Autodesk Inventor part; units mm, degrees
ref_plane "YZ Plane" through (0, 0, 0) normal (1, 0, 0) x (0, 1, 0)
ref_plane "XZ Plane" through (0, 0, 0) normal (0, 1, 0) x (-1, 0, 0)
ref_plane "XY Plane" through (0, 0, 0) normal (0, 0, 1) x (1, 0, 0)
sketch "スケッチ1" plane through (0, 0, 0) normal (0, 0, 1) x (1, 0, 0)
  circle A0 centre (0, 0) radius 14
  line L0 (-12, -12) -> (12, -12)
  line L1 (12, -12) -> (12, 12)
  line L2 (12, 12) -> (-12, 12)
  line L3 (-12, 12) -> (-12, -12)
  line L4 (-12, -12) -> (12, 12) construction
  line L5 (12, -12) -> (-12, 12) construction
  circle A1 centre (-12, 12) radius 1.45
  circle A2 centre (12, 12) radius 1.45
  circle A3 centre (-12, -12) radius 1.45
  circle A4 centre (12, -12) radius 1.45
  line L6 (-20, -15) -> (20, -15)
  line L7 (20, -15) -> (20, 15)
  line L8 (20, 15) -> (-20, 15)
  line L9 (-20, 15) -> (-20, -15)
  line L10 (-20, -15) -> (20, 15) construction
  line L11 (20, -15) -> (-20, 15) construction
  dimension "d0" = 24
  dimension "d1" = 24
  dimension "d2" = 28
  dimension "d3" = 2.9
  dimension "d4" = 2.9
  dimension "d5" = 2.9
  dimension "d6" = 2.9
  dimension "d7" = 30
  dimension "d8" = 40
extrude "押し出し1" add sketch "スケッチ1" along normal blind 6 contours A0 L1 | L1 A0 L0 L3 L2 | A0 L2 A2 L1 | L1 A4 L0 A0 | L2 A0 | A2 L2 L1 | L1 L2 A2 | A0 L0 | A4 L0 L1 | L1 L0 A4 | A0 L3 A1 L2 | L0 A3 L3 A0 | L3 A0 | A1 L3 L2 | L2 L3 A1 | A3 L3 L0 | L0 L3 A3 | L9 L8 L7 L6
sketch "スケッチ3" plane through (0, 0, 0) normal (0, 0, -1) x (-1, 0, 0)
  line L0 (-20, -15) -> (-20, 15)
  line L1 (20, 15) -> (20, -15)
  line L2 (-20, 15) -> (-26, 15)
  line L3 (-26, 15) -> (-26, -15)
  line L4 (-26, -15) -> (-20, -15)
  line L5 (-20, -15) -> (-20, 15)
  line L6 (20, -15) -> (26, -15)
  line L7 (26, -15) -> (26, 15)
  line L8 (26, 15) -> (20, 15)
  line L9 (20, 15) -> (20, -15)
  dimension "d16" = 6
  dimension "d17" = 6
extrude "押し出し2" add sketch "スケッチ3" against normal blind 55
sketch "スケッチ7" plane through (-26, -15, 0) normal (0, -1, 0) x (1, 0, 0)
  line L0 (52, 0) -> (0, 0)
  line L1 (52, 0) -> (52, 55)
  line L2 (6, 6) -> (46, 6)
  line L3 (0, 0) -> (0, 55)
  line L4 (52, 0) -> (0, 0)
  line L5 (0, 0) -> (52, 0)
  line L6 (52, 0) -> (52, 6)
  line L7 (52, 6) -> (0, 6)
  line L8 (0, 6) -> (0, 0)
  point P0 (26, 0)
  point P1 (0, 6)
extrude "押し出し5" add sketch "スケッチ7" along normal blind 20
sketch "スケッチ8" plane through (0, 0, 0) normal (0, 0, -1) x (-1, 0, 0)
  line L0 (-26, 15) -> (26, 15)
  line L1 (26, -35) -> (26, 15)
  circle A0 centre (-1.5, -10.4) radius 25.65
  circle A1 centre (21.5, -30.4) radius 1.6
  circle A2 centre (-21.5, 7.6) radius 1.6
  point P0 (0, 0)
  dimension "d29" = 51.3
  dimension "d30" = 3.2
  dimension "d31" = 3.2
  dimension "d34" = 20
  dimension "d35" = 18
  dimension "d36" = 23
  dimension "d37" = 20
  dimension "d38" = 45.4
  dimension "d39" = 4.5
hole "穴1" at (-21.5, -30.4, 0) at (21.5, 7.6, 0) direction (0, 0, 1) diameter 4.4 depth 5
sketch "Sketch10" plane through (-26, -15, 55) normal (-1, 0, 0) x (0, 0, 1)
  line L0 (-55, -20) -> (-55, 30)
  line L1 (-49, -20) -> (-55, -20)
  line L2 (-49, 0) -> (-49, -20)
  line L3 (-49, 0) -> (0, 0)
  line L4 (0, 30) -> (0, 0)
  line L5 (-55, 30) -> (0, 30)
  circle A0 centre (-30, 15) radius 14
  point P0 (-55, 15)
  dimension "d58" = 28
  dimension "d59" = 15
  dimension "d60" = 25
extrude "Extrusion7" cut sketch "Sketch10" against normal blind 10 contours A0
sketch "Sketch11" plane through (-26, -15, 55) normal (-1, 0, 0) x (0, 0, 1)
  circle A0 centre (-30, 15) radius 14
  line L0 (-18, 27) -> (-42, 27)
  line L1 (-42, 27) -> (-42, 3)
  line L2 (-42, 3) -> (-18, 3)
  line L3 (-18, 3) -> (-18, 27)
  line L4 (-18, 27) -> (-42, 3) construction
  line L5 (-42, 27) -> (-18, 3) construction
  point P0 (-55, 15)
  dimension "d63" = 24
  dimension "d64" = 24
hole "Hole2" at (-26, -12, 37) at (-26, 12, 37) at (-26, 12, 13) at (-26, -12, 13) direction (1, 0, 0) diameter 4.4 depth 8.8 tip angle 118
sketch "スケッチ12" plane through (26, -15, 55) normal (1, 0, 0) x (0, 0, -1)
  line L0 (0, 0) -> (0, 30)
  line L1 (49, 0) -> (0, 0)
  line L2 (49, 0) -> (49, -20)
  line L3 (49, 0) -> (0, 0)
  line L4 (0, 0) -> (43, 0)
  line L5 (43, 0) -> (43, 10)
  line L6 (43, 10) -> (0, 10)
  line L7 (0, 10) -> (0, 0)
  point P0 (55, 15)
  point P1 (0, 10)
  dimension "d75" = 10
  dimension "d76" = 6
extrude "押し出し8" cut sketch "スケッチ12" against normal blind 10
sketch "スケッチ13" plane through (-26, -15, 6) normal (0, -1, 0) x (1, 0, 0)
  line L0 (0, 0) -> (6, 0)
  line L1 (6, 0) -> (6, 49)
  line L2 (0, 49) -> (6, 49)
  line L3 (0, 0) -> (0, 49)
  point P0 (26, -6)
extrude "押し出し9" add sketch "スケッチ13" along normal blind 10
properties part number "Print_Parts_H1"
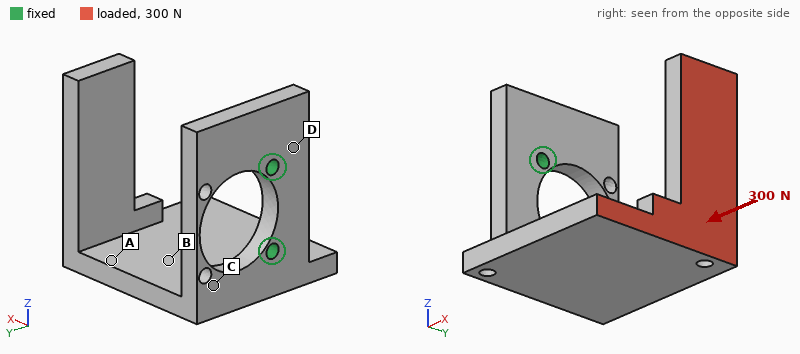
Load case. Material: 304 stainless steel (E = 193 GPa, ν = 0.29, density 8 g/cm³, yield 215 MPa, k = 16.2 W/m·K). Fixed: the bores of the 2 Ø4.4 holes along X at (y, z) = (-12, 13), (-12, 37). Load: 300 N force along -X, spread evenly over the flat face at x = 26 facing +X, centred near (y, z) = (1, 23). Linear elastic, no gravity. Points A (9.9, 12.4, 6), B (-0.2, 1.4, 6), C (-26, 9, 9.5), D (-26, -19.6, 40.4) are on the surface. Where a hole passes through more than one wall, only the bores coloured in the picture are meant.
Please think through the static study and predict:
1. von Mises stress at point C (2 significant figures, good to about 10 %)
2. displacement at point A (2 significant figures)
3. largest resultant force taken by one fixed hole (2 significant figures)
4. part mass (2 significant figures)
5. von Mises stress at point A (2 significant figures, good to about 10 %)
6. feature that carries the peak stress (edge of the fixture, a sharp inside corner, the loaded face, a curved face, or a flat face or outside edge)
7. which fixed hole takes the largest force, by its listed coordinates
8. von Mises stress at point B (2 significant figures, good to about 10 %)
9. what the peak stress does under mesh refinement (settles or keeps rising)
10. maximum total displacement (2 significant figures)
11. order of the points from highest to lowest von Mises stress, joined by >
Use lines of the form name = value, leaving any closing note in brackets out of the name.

von Mises stress at point C = 8.8 MPa
displacement at point A = 0.037 mm
largest resultant force taken by one fixed hole = 250 N
part mass = 240 g
von Mises stress at point A = 28 MPa
feature that carries the peak stress = edge of the fixture
which fixed hole takes the largest force, by its listed coordinates = (-12, 13)
von Mises stress at point B = 23 MPa
what the peak stress does under mesh refinement = keeps rising
maximum total displacement = 0.19 mm
order of the points from highest to lowest von Mises stress, joined by > = A > B > C > D
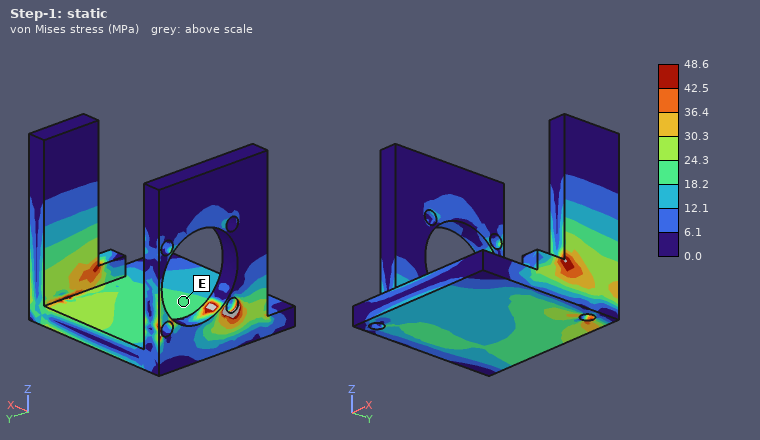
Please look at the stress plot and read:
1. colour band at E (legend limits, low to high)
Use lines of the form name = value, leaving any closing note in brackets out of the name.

colour band at E = 18.2 to 24.3 MPa
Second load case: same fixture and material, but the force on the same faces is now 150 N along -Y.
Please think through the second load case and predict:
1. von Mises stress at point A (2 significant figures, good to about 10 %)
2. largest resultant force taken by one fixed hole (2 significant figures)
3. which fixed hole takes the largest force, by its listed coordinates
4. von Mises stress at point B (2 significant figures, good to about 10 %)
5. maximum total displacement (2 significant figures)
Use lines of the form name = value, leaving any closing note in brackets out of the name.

von Mises stress at point A = 9.1 MPa
largest resultant force taken by one fixed hole = 120 N
which fixed hole takes the largest force, by its listed coordinates = (-12, 13)
von Mises stress at point B = 12 MPa
maximum total displacement = 75 µm
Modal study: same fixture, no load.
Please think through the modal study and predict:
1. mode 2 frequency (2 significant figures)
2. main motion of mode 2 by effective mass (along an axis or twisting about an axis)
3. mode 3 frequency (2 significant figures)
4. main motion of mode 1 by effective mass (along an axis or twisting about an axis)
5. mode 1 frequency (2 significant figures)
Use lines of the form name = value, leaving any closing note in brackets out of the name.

mode 2 frequency = 960 Hz
main motion of mode 2 by effective mass = along Y
mode 3 frequency = 1600 Hz
main motion of mode 1 by effective mass = along Z
mode 1 frequency = 670 Hz
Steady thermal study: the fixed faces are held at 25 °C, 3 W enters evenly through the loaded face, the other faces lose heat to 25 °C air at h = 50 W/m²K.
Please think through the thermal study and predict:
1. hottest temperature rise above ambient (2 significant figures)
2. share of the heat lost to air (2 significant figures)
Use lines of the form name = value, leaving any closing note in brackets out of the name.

hottest temperature rise above ambient = 19 K
share of the heat lost to air = 91 %
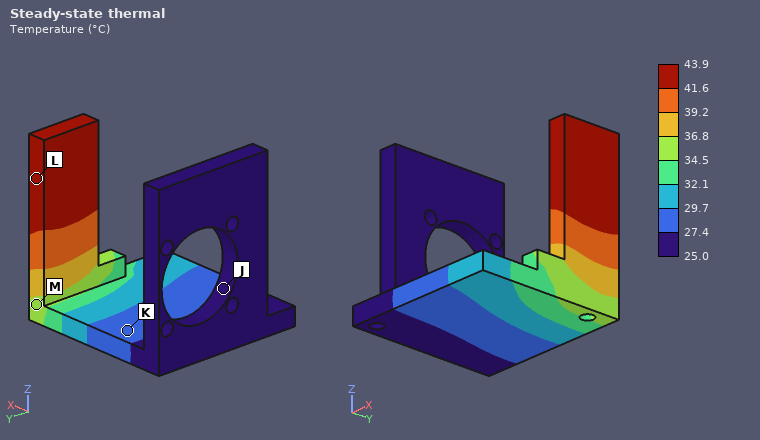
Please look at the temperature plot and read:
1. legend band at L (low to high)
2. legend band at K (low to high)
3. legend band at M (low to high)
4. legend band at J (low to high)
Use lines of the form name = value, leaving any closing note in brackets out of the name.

legend band at L = 41.6 to 43.9 °C
legend band at K = 27.4 to 29.7 °C
legend band at M = 34.5 to 36.8 °C
legend band at J = 25.0 to 27.4 °C
